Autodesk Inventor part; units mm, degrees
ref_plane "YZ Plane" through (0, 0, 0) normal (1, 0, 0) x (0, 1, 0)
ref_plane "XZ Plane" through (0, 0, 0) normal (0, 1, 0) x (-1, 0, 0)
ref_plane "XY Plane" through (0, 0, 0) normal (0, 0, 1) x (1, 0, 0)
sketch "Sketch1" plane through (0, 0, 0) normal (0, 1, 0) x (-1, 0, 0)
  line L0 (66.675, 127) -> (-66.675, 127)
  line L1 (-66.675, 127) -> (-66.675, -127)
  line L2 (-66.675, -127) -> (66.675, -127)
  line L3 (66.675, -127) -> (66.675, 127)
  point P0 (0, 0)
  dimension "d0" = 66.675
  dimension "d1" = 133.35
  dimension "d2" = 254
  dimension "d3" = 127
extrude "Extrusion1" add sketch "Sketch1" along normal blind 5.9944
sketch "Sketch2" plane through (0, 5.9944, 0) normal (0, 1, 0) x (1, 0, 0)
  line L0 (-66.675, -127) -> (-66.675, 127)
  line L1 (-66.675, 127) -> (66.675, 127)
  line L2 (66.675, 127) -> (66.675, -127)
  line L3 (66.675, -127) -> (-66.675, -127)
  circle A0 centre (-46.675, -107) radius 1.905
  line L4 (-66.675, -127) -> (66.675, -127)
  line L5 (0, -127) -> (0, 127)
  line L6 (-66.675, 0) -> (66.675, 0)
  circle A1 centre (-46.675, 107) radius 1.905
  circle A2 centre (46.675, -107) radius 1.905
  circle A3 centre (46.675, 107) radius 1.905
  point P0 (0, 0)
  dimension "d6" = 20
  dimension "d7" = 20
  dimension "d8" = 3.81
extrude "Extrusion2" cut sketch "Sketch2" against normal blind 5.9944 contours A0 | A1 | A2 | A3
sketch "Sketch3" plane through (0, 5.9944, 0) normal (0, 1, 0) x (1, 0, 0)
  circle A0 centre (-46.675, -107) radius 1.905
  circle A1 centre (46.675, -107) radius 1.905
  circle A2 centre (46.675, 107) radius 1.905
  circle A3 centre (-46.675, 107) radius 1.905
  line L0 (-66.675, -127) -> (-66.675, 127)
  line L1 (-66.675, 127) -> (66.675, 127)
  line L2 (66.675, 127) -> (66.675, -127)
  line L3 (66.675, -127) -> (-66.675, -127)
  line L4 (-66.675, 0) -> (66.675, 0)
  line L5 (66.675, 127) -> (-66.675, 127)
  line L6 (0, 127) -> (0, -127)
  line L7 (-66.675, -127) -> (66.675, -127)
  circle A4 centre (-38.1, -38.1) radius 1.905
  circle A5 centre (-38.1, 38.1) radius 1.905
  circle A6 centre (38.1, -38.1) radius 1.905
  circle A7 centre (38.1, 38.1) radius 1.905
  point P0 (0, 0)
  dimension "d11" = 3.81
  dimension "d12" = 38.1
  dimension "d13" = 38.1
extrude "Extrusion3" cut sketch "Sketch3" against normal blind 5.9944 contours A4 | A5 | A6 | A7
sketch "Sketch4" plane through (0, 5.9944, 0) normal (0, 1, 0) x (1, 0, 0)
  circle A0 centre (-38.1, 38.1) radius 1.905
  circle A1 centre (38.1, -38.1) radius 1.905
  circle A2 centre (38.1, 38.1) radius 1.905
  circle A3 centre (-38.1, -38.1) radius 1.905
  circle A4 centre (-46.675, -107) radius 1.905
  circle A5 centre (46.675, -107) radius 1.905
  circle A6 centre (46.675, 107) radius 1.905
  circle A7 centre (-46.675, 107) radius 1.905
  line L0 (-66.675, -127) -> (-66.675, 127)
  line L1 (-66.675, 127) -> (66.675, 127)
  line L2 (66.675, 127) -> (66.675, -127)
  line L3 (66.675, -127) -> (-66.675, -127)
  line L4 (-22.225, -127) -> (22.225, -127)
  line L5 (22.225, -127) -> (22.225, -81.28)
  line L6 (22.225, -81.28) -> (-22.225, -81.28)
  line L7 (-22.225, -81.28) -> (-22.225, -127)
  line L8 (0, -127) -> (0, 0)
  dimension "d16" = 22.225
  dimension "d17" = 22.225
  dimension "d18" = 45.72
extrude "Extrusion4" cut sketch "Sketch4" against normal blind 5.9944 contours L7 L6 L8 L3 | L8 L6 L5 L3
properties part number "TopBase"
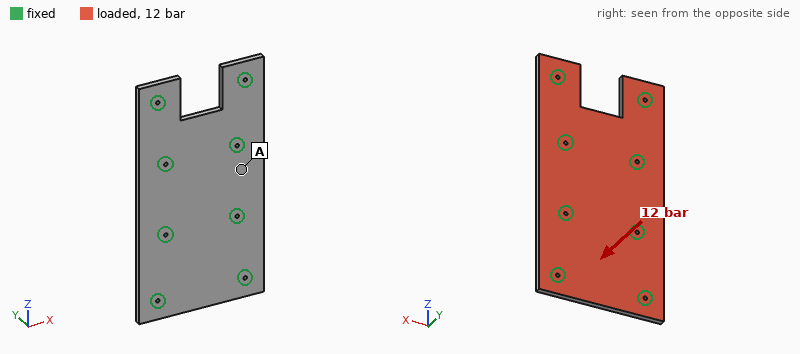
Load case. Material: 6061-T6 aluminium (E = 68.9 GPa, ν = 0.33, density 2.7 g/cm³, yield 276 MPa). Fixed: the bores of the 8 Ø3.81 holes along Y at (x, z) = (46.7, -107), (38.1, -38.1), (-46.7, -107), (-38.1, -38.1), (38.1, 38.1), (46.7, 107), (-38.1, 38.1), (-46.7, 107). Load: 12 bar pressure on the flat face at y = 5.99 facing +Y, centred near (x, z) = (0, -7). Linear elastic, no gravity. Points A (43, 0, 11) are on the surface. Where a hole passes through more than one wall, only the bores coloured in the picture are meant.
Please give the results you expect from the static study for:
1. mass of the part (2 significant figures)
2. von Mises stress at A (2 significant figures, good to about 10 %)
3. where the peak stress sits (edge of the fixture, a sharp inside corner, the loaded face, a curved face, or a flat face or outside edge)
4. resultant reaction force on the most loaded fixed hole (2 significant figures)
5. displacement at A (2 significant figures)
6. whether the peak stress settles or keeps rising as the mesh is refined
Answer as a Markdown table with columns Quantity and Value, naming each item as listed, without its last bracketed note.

| Quantity | Value |
|---|---|
| mass of the part | 510 g |
| von Mises stress at A | 52 MPa |
| where the peak stress sits | edge of the fixture |
| resultant reaction force on the most loaded fixed hole | 6.0 kN |
| displacement at A | 0.10 mm |
| whether the peak stress settles or keeps rising as the mesh is refined | keeps rising |
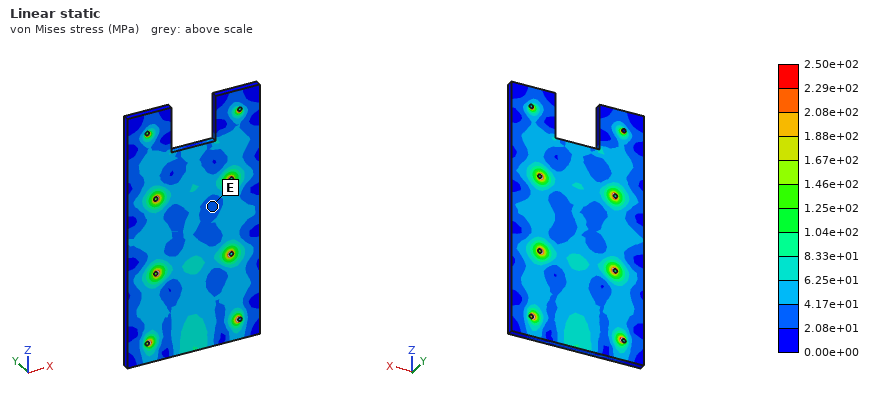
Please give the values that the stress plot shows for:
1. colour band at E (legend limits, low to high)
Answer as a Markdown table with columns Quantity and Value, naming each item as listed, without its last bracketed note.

| Quantity | Value |
|---|---|
| colour band at E | 2.08e+01 to 4.17e+01 MPa |
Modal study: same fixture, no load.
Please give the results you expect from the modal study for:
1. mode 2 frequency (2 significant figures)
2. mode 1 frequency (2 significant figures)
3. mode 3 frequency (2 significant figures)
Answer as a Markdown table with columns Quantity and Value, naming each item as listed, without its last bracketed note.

| Quantity | Value |
|---|---|
| mode 2 frequency | 3300 Hz |
| mode 1 frequency | 2900 Hz |
| mode 3 frequency | 3600 Hz |
